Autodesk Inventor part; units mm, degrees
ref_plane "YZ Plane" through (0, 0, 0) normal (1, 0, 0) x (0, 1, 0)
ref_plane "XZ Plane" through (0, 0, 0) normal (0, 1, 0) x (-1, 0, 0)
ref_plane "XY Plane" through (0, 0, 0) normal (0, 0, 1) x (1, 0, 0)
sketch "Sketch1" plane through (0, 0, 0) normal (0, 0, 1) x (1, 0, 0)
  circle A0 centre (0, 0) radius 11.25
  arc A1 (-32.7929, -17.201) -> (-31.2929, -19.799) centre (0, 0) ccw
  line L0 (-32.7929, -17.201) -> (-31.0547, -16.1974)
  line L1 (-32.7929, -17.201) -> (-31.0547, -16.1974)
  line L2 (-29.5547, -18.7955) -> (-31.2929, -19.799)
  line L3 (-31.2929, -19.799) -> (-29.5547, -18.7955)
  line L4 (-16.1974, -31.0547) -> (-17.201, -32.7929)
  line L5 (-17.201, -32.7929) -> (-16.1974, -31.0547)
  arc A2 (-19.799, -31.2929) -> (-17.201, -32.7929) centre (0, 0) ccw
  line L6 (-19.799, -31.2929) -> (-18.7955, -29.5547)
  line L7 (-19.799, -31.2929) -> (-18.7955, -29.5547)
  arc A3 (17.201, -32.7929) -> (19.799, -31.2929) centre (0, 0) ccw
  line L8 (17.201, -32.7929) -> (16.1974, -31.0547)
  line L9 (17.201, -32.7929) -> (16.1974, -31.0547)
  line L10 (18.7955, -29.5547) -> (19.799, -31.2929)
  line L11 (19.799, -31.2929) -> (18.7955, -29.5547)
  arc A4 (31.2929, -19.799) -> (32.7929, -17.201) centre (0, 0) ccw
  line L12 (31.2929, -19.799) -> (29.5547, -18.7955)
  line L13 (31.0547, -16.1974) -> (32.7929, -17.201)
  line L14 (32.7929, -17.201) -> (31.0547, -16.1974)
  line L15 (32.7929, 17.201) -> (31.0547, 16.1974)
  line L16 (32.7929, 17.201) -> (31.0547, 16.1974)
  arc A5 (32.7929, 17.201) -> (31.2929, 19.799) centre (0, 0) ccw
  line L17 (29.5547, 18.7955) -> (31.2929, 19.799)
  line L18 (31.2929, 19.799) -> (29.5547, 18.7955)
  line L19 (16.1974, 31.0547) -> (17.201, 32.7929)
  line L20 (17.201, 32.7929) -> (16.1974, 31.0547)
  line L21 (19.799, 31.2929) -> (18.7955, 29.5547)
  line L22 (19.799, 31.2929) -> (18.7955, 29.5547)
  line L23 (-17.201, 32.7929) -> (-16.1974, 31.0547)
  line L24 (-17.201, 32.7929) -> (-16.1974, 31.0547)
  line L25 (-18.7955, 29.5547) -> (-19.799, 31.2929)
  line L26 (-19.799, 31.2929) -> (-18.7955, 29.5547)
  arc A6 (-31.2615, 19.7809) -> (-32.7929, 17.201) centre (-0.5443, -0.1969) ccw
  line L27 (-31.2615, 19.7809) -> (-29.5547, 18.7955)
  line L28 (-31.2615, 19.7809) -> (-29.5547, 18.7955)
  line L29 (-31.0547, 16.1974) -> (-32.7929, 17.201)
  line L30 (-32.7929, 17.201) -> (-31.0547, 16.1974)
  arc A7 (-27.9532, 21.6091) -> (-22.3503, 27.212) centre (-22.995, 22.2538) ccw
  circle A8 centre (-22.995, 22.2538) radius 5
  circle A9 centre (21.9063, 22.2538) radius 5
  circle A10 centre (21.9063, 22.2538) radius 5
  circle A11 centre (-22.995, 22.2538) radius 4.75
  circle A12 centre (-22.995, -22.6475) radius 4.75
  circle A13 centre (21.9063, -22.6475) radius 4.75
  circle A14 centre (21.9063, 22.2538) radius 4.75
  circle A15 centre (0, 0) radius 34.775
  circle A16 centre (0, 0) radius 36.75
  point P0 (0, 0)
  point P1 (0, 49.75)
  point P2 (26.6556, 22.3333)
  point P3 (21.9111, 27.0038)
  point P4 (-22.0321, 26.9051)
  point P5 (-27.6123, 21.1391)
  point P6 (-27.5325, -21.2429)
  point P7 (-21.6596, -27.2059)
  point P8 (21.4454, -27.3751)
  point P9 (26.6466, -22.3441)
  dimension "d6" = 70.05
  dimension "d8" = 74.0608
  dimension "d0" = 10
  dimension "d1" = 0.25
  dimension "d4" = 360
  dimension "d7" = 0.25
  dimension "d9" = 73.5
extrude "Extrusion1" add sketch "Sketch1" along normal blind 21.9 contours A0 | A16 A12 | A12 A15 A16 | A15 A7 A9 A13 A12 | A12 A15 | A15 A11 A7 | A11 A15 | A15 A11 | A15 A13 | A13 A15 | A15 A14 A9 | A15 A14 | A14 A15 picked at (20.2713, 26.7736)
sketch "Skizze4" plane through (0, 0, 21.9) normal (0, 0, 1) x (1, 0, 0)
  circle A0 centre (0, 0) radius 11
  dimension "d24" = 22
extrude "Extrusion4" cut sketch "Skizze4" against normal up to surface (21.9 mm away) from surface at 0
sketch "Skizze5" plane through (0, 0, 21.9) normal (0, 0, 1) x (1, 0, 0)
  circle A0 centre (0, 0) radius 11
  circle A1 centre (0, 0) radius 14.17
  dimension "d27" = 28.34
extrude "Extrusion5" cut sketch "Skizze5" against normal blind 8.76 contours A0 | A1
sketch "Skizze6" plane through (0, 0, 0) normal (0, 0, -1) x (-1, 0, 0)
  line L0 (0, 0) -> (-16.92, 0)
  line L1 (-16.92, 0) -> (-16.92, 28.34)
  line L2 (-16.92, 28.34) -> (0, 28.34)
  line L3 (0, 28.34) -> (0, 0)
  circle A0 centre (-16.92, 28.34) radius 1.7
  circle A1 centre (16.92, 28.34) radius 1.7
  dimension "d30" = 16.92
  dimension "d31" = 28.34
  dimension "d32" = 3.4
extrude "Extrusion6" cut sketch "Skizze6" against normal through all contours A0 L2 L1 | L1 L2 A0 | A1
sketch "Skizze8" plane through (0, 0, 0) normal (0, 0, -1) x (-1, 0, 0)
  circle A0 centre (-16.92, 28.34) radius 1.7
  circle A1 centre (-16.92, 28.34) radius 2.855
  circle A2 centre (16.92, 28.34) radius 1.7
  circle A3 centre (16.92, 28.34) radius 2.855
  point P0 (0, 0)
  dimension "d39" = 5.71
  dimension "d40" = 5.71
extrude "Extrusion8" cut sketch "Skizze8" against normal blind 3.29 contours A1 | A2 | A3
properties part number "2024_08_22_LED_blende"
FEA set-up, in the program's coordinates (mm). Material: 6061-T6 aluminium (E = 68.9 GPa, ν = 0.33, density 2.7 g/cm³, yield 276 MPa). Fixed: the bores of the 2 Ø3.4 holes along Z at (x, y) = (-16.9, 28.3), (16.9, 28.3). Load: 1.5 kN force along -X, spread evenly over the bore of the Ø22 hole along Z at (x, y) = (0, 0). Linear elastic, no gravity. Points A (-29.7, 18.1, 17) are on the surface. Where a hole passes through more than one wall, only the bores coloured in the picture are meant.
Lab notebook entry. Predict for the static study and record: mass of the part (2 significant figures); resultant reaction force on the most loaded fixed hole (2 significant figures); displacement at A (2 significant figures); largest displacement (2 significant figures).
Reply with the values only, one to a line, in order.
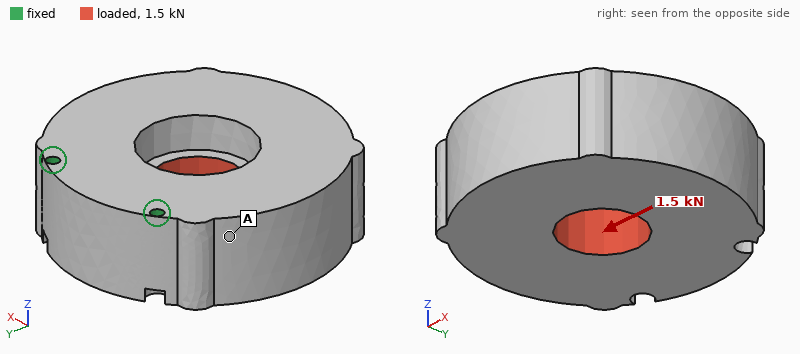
200 g
1.4 kN
3.3 µm
8.9 µm
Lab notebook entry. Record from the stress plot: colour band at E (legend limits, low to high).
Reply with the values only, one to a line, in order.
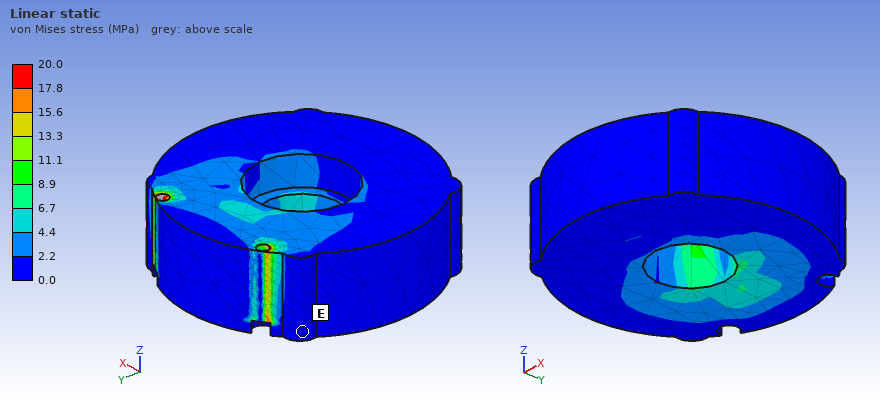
0.0 to 2.2 MPa
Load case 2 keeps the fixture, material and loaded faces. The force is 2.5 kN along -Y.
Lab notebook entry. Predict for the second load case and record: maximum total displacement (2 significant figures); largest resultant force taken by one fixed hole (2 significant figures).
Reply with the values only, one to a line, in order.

12 µm
1.3 kN
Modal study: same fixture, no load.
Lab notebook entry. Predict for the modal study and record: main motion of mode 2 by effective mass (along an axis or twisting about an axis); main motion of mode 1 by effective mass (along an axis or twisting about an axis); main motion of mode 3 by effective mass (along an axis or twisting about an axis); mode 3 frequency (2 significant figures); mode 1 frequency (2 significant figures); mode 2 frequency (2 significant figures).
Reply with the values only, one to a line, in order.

along X
along Z
twisting about Y
7300 Hz
3000 Hz
5100 Hz
